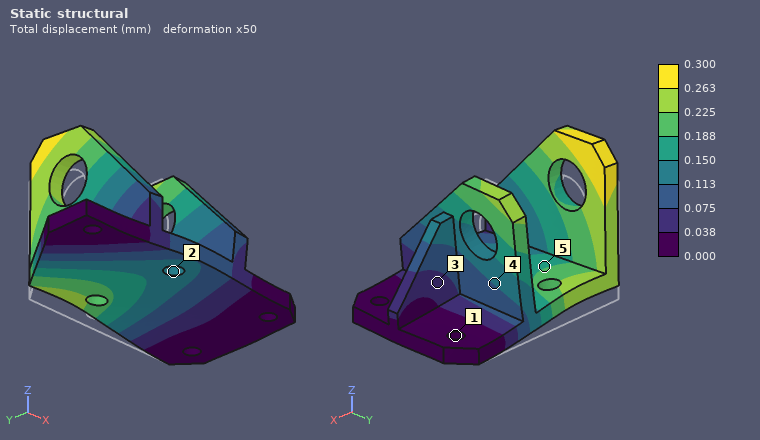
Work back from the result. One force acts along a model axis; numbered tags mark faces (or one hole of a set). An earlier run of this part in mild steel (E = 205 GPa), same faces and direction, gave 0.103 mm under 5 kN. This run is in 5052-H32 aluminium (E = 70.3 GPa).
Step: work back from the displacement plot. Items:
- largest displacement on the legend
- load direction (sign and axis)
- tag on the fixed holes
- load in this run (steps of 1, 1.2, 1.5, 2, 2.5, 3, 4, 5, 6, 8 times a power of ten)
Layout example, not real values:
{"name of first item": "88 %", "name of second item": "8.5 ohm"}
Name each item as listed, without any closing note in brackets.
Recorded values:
{"largest displacement on the legend": "0.300 mm", "load direction": "+Z", "tag on the fixed holes": "1", "load in this run": "5 kN"}
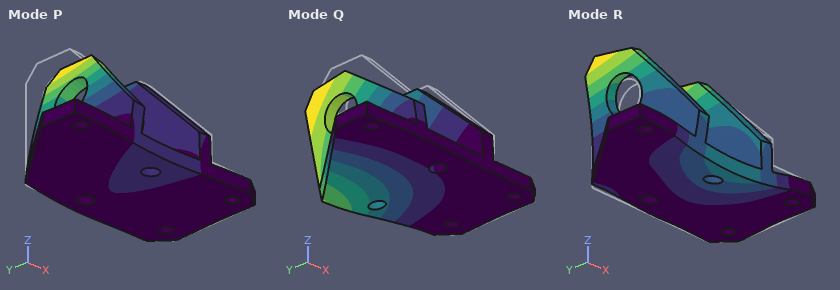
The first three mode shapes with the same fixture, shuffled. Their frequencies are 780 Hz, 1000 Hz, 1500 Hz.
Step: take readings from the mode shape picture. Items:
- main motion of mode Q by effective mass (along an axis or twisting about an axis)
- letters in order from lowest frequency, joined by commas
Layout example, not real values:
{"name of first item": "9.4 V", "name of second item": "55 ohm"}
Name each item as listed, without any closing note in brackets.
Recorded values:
{"main motion of mode Q by effective mass": "along Z", "letters in order from lowest frequency, joined by commas": "Q, P, R"}
